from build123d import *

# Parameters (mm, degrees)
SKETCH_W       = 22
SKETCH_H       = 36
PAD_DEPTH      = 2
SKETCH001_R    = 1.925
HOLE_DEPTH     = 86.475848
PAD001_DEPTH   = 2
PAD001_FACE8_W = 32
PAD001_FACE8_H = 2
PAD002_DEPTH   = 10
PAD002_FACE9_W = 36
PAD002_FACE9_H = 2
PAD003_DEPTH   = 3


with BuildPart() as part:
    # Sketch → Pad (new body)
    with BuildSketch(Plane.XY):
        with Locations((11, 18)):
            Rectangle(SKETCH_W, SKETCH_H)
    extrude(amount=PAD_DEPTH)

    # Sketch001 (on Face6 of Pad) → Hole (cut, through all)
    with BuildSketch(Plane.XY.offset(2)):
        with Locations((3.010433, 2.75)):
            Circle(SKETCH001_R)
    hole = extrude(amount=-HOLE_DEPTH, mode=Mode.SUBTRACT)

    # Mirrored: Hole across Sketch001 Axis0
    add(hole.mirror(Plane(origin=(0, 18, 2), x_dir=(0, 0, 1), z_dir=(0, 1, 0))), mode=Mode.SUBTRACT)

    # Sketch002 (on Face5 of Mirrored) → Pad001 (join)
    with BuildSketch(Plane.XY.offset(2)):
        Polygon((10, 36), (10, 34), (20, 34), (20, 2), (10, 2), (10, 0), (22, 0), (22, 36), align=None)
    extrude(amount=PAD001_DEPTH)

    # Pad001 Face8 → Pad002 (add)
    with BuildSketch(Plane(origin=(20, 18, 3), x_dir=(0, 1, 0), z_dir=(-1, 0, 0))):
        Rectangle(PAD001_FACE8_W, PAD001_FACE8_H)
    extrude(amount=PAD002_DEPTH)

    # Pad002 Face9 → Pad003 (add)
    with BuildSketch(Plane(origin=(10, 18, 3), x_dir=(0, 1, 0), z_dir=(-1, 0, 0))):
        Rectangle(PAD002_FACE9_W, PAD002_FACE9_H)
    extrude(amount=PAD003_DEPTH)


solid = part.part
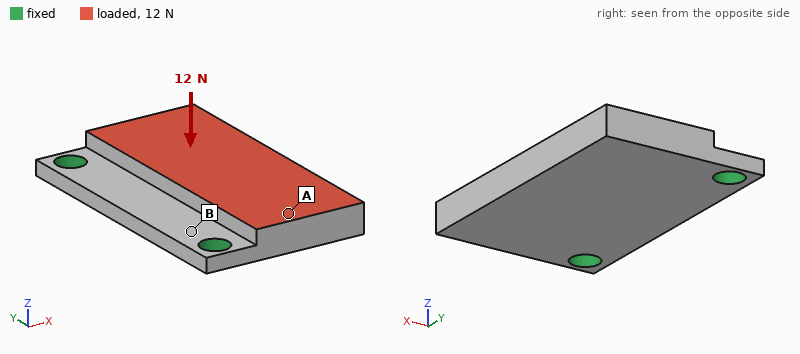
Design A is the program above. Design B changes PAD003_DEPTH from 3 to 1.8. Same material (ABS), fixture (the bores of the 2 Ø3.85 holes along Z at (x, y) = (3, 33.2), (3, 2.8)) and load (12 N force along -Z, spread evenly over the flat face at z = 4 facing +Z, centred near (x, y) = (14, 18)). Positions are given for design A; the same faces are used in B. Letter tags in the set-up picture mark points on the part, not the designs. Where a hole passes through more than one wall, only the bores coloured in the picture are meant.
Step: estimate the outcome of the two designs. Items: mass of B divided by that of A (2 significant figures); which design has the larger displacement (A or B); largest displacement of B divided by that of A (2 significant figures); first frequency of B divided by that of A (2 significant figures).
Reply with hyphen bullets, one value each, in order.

- 0.97
- B
- 1.2
- 0.95
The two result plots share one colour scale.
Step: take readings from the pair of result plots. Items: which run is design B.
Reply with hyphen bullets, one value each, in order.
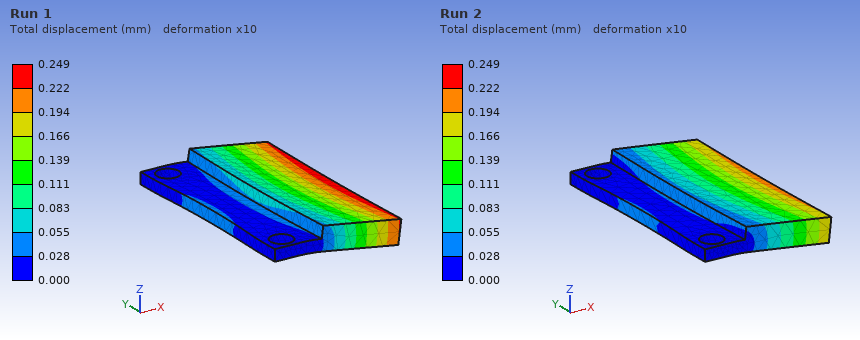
- Run 1
